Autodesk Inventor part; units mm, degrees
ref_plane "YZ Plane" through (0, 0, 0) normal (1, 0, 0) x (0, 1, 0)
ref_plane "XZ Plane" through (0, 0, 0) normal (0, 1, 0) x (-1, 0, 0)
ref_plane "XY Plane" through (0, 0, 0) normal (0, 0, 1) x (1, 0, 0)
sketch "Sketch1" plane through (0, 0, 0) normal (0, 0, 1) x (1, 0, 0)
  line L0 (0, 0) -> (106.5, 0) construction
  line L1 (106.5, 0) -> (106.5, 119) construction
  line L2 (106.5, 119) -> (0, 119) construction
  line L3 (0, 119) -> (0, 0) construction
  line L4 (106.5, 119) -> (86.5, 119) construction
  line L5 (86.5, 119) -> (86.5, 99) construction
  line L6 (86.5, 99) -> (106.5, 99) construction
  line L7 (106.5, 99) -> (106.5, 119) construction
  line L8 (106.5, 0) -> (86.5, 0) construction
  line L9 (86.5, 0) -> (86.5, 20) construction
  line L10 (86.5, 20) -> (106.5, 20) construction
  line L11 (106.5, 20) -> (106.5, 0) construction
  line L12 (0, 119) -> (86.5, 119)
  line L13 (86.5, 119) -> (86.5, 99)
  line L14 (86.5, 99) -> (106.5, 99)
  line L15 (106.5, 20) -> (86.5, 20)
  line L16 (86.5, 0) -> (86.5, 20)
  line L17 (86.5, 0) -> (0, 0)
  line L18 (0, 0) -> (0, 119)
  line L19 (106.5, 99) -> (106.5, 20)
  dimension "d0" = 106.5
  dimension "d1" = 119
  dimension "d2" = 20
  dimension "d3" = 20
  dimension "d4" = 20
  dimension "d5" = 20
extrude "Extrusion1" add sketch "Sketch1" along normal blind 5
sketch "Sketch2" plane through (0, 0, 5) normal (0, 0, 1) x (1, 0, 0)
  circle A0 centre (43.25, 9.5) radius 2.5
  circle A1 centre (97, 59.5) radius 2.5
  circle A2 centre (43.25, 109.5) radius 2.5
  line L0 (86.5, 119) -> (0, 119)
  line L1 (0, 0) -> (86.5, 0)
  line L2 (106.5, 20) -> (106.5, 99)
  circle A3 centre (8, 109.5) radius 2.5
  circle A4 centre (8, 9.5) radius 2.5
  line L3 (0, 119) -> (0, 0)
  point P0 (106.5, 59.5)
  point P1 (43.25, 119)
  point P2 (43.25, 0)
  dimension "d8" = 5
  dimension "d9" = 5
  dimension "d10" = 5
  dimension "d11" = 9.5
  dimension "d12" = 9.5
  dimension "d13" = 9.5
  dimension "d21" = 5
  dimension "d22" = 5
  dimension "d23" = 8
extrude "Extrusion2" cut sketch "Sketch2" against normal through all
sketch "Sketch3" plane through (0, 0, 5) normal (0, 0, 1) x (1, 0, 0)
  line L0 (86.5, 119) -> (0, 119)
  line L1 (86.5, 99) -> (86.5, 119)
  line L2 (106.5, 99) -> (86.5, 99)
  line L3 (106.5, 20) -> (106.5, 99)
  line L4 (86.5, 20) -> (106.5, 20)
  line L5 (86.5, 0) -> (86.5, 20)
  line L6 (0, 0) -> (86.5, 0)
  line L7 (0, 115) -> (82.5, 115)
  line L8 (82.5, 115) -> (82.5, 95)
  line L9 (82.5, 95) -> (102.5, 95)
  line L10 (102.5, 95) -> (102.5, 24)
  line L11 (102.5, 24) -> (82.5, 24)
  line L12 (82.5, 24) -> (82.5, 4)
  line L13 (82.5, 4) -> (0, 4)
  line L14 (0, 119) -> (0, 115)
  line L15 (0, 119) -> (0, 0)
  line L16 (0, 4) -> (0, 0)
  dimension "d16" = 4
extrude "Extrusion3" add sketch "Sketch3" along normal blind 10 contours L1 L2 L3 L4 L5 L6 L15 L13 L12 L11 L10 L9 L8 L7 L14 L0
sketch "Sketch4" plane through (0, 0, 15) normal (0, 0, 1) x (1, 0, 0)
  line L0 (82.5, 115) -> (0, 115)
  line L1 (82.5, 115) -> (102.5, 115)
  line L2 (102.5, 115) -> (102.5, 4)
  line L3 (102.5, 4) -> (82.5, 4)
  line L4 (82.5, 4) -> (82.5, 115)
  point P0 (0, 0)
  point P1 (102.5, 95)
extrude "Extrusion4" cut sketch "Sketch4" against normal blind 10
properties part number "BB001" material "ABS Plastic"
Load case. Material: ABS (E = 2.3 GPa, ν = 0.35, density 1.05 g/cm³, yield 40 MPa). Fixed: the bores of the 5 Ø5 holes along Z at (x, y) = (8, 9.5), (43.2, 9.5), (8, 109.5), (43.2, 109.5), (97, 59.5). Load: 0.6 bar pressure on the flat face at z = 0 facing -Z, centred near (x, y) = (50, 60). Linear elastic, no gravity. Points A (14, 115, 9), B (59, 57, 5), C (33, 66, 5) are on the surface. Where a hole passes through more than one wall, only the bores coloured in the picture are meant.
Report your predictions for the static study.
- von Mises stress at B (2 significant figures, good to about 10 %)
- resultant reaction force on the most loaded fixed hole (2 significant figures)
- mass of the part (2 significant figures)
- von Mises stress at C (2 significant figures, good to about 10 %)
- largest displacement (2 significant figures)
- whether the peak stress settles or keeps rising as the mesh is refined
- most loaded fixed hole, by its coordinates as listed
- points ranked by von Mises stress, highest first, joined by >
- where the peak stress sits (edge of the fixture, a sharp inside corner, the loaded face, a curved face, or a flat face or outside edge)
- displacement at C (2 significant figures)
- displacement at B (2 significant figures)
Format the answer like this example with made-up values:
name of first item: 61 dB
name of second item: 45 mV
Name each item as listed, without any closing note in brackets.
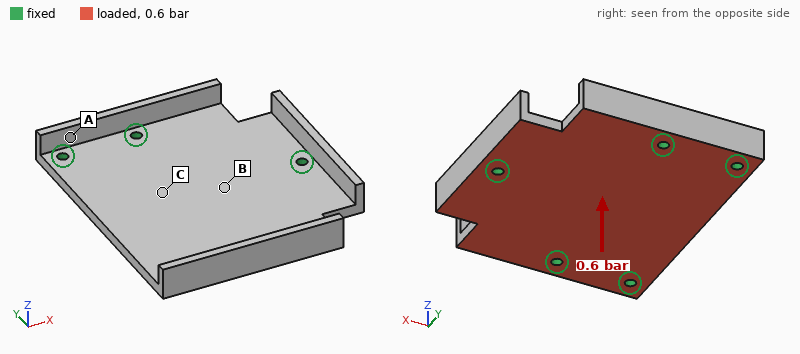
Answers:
von Mises stress at B: 3.3 MPa
resultant reaction force on the most loaded fixed hole: 200 N
mass of the part: 72 g
von Mises stress at C: 4.7 MPa
largest displacement: 0.73 mm
whether the peak stress settles or keeps rising as the mesh is refined: keeps rising
most loaded fixed hole, by its coordinates as listed: (97, 59.5)
points ranked by von Mises stress, highest first, joined by >: C > B > A
where the peak stress sits: edge of the fixture
displacement at C: 0.58 mm
displacement at B: 0.45 mm
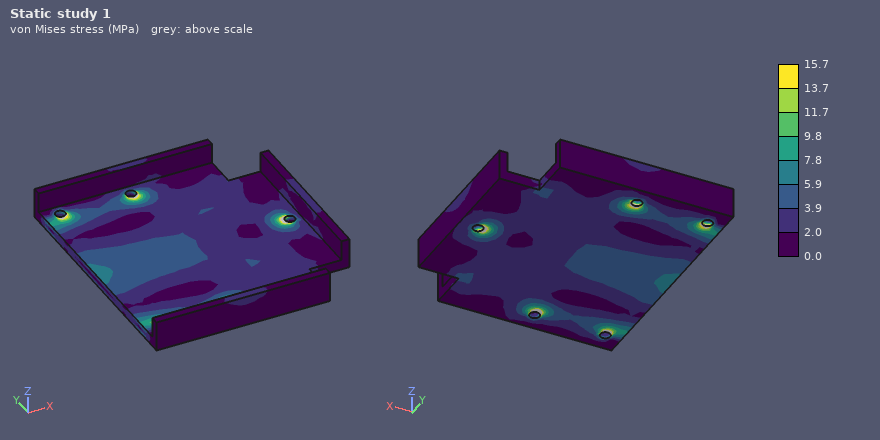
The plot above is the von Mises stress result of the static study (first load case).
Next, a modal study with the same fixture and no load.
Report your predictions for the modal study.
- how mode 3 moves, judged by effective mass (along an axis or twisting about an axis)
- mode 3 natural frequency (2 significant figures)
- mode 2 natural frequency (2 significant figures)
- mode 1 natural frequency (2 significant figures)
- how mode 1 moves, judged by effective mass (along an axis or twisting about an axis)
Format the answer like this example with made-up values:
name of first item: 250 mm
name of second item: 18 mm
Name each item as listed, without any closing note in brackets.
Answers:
how mode 3 moves, judged by effective mass: along Z
mode 3 natural frequency: 1200 Hz
mode 2 natural frequency: 1000 Hz
mode 1 natural frequency: 800 Hz
how mode 1 moves, judged by effective mass: along Z
